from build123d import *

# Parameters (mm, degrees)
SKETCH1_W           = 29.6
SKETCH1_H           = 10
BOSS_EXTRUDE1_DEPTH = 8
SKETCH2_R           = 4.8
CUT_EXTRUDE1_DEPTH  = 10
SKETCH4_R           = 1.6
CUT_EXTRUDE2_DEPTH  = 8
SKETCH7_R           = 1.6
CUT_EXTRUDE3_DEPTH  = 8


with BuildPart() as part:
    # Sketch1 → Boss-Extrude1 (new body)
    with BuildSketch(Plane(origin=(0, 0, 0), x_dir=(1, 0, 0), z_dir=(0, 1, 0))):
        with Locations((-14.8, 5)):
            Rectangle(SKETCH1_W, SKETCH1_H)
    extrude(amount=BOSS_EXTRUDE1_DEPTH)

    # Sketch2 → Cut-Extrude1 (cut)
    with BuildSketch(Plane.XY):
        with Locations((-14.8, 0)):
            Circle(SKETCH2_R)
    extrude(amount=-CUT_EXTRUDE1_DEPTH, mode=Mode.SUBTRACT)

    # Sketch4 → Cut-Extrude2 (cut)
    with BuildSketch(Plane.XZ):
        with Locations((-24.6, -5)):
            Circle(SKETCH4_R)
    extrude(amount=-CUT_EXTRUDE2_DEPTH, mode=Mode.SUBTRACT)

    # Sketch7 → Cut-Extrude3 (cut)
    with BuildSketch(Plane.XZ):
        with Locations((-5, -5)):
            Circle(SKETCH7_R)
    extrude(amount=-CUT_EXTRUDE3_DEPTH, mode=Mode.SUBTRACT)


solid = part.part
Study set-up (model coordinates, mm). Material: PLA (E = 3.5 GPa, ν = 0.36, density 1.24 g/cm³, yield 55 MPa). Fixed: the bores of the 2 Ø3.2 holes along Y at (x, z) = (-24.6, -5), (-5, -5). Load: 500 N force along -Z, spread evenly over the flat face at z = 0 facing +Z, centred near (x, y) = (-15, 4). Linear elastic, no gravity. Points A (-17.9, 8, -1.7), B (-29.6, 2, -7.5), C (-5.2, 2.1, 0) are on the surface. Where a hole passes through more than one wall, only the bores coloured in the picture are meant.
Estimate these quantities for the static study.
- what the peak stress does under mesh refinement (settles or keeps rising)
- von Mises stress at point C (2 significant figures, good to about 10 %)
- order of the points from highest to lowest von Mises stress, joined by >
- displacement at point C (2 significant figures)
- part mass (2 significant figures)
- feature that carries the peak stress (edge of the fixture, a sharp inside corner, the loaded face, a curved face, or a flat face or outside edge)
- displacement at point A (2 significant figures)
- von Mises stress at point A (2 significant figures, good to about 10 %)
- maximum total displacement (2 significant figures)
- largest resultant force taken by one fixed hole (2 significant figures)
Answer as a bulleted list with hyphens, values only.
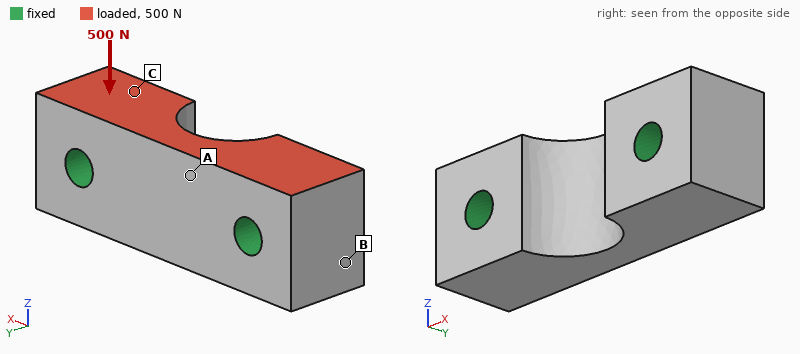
- keeps rising
- 4.5 MPa
- C > A > B
- 4.0 µm
- 2.3 g
- edge of the fixture
- 13 µm
- 2.7 MPa
- 17 µm
- 250 N
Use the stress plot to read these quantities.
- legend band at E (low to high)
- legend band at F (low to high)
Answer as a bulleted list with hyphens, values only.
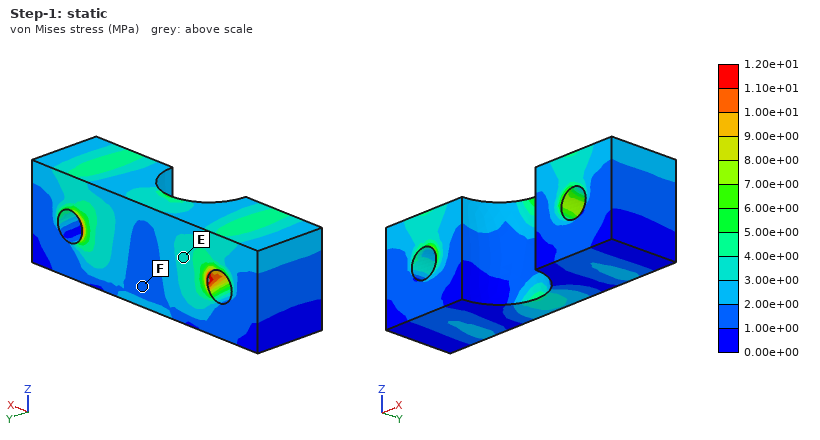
- 3.00e+00 to 4.00e+00 MPa
- 1.00e+00 to 2.00e+00 MPa
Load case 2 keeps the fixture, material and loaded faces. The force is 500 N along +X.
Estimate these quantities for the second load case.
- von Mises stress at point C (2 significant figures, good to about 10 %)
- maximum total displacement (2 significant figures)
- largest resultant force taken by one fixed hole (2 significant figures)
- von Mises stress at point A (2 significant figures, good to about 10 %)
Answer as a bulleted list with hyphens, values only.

- 4.6 MPa
- 24 µm
- 260 N
- 4.4 MPa
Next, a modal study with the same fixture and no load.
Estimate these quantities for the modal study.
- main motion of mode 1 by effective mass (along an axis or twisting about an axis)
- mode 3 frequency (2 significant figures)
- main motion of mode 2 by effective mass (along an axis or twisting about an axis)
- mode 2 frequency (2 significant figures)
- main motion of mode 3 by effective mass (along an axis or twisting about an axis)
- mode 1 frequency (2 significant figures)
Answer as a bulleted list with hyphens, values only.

- along Z
- 30 kHz
- along Y
- 24 kHz
- twisting about X
- 20 kHz
